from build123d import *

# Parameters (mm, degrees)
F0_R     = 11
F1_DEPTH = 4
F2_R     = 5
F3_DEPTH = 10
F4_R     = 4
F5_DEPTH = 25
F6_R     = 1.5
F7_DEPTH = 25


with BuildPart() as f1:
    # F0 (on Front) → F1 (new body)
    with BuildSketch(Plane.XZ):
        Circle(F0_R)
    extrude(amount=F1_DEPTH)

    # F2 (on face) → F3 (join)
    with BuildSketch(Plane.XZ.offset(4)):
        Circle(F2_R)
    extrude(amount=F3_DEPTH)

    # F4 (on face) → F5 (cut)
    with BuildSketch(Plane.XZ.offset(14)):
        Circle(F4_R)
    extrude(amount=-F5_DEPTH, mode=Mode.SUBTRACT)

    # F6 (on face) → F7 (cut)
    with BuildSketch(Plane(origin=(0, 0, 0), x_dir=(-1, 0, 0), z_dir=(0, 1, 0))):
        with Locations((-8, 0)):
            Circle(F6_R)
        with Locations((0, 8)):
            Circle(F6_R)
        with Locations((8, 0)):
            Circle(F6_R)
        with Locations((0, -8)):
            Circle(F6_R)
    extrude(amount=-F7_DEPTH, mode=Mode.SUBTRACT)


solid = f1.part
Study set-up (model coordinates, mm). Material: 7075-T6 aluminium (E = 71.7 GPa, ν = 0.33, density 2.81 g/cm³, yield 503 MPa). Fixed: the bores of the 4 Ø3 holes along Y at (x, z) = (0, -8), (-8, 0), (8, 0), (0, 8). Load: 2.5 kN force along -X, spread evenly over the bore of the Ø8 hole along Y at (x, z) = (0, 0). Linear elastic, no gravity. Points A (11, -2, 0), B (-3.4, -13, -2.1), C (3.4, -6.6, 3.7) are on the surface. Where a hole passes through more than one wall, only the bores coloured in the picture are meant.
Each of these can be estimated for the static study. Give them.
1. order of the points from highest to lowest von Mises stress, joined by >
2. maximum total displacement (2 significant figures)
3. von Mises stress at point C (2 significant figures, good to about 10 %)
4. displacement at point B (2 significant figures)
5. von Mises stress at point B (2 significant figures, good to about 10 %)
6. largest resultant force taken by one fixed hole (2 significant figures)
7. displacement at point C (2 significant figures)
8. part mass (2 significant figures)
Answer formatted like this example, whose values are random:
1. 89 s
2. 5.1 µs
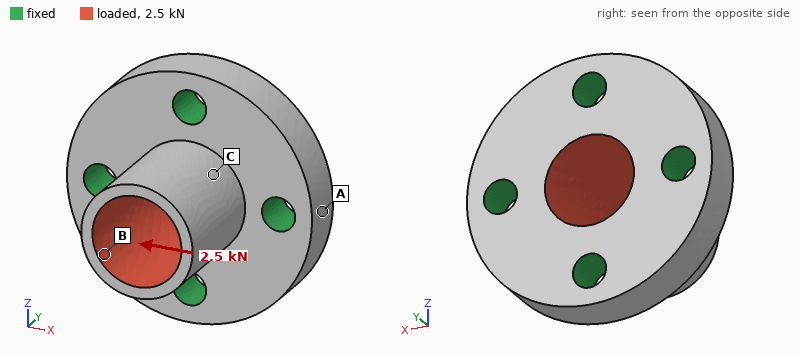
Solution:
1. C > B > A
2. 50 µm
3. 100 MPa
4. 46 µm
5. 35 MPa
6. 1.1 kN
7. 19 µm
8. 4.2 g
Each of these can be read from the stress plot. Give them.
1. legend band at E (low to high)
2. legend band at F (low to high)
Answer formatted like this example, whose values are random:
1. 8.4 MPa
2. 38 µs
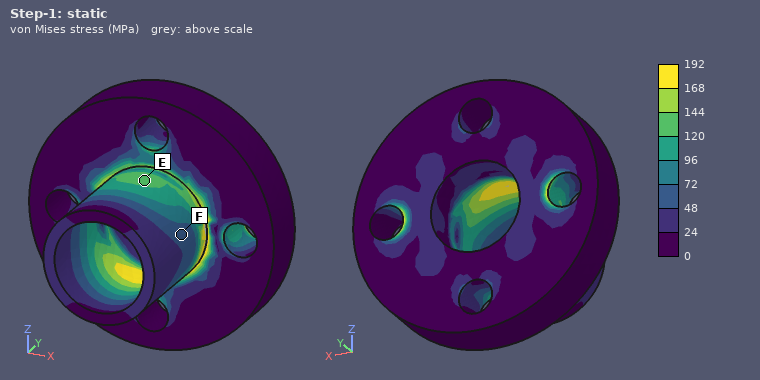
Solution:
1. 120 to 144 MPa
2. 48 to 72 MPa
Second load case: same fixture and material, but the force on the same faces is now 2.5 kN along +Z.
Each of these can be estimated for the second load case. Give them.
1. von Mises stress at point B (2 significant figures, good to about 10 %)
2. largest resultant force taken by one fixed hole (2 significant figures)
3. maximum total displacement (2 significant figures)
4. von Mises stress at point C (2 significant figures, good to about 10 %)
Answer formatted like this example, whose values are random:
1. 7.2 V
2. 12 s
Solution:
1. 33 MPa
2. 1.1 kN
3. 50 µm
4. 98 MPa
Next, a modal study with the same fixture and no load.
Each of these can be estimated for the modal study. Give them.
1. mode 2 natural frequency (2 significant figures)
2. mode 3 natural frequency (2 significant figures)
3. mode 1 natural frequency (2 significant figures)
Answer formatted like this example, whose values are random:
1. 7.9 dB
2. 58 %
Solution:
1. 39 kHz
2. 40 kHz
3. 39 kHz
